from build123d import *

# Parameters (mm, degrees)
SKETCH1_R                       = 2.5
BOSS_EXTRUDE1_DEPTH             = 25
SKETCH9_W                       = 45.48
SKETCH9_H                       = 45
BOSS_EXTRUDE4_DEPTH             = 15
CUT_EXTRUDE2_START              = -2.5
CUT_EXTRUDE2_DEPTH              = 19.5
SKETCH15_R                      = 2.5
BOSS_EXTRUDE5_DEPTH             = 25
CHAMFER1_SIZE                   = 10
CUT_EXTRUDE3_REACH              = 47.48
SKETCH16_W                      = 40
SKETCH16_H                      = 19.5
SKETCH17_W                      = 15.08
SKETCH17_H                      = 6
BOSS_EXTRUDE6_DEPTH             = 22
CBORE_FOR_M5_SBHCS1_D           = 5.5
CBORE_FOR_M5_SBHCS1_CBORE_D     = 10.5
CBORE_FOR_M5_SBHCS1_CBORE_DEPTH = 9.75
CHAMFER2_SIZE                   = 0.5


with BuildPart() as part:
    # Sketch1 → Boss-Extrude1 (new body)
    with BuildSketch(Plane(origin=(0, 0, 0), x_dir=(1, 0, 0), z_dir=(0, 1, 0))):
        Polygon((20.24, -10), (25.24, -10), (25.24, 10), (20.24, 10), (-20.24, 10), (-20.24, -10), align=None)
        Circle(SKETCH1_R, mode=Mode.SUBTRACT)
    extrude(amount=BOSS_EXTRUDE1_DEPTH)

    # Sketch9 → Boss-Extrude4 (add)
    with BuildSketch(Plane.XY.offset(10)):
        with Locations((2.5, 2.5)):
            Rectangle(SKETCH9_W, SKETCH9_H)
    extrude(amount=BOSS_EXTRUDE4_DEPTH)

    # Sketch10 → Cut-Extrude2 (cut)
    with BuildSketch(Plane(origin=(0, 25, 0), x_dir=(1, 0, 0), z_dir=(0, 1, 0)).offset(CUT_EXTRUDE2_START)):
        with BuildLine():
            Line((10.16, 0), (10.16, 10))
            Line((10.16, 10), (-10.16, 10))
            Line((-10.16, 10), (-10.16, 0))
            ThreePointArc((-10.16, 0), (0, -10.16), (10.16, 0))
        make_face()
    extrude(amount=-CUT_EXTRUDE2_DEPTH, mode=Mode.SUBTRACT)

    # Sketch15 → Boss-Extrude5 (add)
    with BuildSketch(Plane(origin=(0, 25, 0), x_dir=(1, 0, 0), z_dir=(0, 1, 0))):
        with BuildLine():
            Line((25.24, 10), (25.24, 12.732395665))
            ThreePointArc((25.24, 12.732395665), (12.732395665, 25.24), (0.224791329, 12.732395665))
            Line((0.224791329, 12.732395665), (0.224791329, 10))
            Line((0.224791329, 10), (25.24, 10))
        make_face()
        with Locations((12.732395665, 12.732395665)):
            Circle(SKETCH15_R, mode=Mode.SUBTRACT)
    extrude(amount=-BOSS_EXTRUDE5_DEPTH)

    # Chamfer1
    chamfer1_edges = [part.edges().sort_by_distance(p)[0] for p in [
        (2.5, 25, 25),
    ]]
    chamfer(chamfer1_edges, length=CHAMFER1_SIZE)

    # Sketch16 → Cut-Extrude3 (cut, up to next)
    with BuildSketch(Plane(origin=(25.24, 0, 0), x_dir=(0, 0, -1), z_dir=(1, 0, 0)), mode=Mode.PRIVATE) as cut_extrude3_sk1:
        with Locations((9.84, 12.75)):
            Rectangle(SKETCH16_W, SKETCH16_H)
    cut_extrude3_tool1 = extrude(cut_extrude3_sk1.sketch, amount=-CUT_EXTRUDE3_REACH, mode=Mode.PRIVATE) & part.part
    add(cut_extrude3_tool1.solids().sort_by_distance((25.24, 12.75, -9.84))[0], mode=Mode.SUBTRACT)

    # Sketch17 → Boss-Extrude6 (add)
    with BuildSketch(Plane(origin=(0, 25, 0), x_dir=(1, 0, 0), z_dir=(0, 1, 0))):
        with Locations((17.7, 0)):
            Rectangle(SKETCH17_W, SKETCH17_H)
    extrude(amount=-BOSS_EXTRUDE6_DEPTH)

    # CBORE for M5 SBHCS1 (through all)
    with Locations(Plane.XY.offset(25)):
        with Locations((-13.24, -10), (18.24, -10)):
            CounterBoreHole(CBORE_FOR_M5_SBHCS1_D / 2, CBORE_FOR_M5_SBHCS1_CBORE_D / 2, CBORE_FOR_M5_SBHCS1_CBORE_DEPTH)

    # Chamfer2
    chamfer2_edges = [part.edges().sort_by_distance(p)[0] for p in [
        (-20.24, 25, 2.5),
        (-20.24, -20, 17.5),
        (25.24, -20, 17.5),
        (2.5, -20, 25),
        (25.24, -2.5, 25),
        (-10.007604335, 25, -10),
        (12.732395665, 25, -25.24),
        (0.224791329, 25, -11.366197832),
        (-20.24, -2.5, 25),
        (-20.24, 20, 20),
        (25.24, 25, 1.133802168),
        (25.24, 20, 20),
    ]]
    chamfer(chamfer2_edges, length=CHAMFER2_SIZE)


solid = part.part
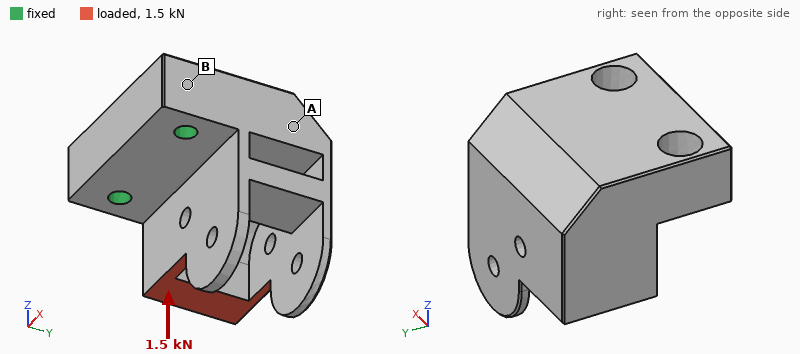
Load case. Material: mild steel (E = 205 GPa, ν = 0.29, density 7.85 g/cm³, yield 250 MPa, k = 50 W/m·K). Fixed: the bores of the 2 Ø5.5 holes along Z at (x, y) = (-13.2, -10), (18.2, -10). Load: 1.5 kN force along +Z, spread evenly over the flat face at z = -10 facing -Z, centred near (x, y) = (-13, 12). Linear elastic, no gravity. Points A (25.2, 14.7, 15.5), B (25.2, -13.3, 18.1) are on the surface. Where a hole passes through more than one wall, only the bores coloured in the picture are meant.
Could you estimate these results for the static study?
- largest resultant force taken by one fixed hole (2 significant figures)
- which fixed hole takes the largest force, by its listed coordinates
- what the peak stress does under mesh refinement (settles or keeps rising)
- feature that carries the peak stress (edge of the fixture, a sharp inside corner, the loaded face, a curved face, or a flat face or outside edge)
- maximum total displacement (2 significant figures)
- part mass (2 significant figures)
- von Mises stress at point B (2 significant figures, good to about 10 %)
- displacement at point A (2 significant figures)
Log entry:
1.5 kN
(-13.2, -10)
keeps rising
edge of the fixture
36 µm
310 g
24 MPa
14 µm
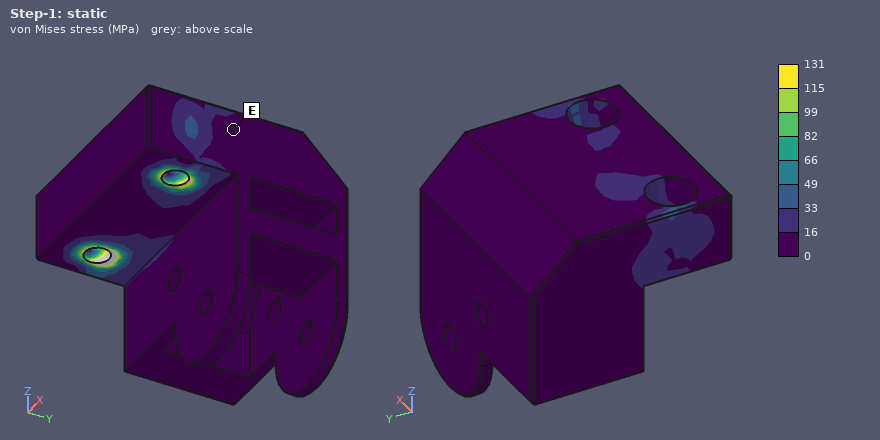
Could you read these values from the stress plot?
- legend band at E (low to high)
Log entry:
0 to 16 MPa
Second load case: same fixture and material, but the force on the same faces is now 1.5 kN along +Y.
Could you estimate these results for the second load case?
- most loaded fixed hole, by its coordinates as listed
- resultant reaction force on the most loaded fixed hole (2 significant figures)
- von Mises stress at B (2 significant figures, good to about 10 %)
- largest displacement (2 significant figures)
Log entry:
(-13.2, -10)
1.5 kN
29 MPa
49 µm
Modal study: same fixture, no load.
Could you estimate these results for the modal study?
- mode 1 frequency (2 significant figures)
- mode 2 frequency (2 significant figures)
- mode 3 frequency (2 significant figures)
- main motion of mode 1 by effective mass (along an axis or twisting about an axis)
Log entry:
2700 Hz
4500 Hz
5100 Hz
along Z
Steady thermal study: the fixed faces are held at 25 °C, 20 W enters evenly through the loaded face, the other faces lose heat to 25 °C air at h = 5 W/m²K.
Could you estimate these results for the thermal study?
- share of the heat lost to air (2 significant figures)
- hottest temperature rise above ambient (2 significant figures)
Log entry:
5.2 %
45 K
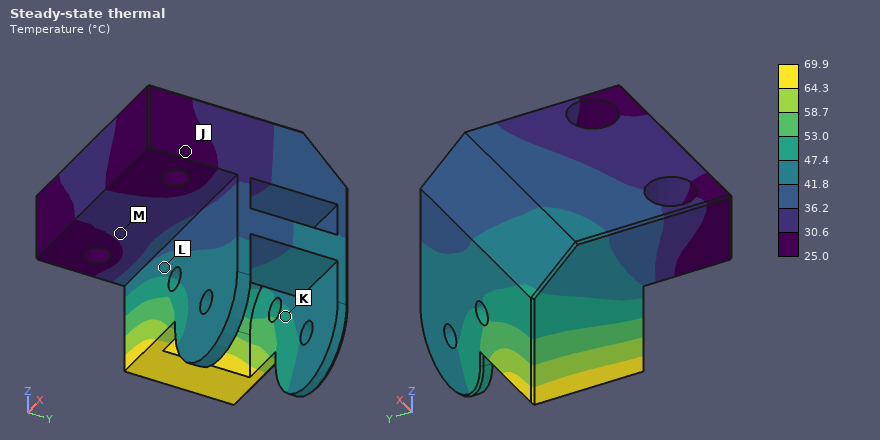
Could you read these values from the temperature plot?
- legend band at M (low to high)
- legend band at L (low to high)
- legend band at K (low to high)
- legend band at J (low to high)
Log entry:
30.6 to 36.2 °C
41.8 to 47.4 °C
47.4 to 53.0 °C
25.0 to 30.6 °C
